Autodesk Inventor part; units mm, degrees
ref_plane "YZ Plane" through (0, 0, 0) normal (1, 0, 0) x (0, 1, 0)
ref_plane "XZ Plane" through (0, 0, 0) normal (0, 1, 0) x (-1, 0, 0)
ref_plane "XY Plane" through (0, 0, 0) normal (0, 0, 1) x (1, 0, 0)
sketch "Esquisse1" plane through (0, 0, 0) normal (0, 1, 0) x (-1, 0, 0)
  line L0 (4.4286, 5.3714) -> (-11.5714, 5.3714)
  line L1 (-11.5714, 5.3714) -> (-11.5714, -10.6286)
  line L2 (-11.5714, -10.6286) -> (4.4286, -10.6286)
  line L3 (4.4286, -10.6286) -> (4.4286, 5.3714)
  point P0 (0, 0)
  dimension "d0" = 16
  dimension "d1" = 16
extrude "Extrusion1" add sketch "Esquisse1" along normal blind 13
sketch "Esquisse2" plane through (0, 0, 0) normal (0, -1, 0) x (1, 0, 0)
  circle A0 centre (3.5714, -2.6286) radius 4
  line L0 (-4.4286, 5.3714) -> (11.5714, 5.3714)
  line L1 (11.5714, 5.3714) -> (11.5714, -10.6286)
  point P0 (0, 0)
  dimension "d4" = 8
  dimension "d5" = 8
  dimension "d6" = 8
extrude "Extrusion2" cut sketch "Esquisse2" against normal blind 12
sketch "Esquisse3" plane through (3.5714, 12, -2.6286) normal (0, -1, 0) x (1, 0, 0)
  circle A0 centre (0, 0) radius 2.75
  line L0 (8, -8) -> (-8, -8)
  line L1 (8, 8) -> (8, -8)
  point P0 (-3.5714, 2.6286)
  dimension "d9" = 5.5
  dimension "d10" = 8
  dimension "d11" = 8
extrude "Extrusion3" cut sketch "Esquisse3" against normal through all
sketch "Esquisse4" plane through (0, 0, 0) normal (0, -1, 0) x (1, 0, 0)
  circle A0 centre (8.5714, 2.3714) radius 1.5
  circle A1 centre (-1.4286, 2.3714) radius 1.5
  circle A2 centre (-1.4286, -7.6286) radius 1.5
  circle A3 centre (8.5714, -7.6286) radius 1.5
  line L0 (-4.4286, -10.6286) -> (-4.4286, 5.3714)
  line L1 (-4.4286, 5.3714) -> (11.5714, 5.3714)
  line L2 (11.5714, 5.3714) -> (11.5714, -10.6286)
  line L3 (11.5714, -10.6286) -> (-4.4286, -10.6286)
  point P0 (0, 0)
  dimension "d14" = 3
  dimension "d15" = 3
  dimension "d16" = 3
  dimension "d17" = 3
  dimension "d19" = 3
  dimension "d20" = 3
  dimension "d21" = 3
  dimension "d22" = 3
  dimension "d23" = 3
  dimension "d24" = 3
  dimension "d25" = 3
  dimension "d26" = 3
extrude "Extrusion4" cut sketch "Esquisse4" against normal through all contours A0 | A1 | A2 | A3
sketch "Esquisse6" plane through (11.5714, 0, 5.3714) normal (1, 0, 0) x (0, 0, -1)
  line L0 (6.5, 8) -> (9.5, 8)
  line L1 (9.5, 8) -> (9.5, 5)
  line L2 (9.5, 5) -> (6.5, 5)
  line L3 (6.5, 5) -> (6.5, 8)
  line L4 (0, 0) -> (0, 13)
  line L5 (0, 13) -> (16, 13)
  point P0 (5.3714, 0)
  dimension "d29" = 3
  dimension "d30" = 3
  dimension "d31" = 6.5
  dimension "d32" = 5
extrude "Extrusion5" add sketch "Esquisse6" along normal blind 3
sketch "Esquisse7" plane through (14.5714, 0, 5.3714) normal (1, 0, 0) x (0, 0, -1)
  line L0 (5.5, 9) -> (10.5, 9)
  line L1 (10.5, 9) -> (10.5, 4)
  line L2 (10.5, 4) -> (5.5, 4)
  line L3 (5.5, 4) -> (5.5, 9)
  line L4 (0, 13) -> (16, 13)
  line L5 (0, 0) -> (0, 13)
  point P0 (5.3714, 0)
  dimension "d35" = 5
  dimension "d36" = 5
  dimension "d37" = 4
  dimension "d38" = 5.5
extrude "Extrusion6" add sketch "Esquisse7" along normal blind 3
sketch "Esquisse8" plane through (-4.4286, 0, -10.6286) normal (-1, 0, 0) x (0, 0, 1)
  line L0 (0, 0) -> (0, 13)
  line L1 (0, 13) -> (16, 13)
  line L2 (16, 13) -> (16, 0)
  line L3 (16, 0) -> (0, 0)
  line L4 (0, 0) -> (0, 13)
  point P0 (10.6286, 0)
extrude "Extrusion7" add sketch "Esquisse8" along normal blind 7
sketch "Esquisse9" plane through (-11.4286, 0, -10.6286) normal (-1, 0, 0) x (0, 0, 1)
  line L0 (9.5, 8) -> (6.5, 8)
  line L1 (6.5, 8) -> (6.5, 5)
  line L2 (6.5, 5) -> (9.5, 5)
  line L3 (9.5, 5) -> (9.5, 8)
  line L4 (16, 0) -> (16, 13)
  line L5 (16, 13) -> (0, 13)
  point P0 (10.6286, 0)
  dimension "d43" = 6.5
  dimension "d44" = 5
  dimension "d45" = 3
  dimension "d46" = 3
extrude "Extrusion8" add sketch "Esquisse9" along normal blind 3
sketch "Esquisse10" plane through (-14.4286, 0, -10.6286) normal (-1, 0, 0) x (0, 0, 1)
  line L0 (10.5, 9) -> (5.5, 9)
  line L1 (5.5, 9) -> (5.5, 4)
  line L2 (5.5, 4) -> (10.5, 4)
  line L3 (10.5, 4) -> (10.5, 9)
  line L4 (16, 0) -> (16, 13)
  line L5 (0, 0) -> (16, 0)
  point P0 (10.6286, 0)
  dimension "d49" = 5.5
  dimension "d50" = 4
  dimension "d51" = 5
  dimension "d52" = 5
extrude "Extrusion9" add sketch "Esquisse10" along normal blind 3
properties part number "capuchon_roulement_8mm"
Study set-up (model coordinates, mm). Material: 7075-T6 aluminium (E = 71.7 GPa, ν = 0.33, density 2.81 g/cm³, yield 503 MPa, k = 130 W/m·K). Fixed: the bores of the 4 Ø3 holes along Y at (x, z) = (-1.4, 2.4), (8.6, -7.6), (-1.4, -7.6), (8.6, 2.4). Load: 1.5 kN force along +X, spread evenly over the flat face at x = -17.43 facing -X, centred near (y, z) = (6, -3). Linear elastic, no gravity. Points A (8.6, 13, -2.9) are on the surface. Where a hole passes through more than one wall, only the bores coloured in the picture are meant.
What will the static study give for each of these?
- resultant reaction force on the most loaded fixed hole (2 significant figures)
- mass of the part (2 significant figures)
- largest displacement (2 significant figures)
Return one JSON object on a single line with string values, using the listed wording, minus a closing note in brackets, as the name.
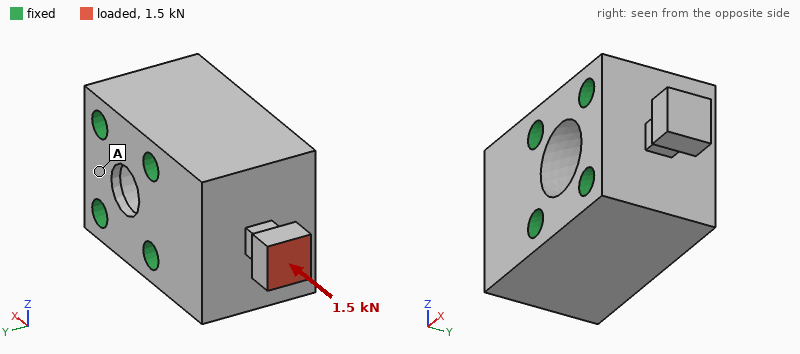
{"resultant reaction force on the most loaded fixed hole": "790 N", "mass of the part": "11 g", "largest displacement": "16 µm"}
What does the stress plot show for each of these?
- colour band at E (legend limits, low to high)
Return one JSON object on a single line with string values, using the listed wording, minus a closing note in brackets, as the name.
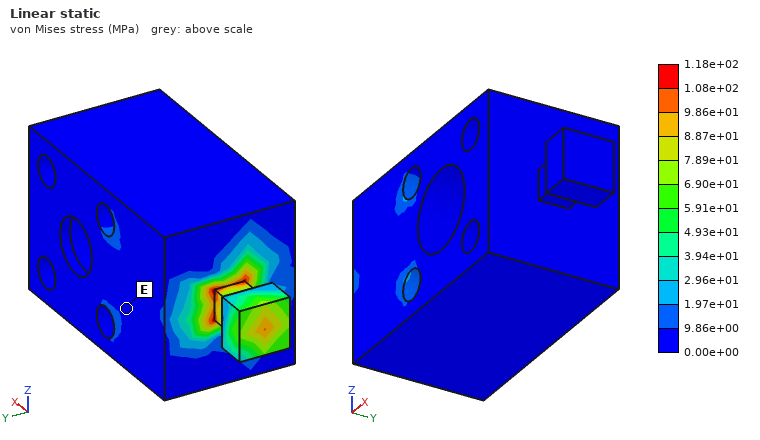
{"colour band at E": "0.00e+00 to 9.86e+00 MPa"}
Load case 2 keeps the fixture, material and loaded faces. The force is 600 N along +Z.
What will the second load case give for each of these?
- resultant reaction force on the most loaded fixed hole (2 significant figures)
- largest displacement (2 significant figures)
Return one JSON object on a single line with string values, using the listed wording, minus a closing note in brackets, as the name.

{"resultant reaction force on the most loaded fixed hole": "850 N", "largest displacement": "0.14 mm"}
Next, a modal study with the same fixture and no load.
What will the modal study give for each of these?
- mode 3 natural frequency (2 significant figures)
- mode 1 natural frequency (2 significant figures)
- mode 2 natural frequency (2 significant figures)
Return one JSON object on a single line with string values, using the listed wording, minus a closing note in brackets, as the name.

{"mode 3 natural frequency": "30 kHz", "mode 1 natural frequency": "30 kHz", "mode 2 natural frequency": "30 kHz"}
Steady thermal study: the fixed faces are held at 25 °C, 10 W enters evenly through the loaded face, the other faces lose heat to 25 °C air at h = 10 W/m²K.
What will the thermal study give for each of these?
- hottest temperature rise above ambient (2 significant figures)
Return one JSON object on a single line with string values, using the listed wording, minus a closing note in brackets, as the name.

{"hottest temperature rise above ambient": "49 K"}
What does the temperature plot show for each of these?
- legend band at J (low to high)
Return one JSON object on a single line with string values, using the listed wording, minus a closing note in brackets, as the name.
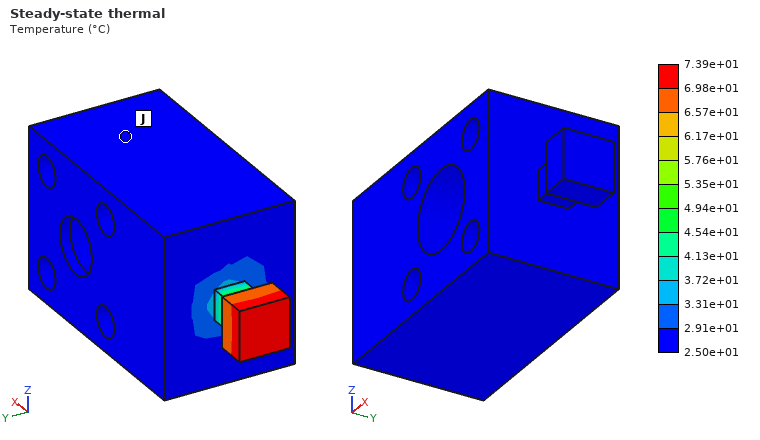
{"legend band at J": "2.50e+01 to 2.91e+01 °C"}
